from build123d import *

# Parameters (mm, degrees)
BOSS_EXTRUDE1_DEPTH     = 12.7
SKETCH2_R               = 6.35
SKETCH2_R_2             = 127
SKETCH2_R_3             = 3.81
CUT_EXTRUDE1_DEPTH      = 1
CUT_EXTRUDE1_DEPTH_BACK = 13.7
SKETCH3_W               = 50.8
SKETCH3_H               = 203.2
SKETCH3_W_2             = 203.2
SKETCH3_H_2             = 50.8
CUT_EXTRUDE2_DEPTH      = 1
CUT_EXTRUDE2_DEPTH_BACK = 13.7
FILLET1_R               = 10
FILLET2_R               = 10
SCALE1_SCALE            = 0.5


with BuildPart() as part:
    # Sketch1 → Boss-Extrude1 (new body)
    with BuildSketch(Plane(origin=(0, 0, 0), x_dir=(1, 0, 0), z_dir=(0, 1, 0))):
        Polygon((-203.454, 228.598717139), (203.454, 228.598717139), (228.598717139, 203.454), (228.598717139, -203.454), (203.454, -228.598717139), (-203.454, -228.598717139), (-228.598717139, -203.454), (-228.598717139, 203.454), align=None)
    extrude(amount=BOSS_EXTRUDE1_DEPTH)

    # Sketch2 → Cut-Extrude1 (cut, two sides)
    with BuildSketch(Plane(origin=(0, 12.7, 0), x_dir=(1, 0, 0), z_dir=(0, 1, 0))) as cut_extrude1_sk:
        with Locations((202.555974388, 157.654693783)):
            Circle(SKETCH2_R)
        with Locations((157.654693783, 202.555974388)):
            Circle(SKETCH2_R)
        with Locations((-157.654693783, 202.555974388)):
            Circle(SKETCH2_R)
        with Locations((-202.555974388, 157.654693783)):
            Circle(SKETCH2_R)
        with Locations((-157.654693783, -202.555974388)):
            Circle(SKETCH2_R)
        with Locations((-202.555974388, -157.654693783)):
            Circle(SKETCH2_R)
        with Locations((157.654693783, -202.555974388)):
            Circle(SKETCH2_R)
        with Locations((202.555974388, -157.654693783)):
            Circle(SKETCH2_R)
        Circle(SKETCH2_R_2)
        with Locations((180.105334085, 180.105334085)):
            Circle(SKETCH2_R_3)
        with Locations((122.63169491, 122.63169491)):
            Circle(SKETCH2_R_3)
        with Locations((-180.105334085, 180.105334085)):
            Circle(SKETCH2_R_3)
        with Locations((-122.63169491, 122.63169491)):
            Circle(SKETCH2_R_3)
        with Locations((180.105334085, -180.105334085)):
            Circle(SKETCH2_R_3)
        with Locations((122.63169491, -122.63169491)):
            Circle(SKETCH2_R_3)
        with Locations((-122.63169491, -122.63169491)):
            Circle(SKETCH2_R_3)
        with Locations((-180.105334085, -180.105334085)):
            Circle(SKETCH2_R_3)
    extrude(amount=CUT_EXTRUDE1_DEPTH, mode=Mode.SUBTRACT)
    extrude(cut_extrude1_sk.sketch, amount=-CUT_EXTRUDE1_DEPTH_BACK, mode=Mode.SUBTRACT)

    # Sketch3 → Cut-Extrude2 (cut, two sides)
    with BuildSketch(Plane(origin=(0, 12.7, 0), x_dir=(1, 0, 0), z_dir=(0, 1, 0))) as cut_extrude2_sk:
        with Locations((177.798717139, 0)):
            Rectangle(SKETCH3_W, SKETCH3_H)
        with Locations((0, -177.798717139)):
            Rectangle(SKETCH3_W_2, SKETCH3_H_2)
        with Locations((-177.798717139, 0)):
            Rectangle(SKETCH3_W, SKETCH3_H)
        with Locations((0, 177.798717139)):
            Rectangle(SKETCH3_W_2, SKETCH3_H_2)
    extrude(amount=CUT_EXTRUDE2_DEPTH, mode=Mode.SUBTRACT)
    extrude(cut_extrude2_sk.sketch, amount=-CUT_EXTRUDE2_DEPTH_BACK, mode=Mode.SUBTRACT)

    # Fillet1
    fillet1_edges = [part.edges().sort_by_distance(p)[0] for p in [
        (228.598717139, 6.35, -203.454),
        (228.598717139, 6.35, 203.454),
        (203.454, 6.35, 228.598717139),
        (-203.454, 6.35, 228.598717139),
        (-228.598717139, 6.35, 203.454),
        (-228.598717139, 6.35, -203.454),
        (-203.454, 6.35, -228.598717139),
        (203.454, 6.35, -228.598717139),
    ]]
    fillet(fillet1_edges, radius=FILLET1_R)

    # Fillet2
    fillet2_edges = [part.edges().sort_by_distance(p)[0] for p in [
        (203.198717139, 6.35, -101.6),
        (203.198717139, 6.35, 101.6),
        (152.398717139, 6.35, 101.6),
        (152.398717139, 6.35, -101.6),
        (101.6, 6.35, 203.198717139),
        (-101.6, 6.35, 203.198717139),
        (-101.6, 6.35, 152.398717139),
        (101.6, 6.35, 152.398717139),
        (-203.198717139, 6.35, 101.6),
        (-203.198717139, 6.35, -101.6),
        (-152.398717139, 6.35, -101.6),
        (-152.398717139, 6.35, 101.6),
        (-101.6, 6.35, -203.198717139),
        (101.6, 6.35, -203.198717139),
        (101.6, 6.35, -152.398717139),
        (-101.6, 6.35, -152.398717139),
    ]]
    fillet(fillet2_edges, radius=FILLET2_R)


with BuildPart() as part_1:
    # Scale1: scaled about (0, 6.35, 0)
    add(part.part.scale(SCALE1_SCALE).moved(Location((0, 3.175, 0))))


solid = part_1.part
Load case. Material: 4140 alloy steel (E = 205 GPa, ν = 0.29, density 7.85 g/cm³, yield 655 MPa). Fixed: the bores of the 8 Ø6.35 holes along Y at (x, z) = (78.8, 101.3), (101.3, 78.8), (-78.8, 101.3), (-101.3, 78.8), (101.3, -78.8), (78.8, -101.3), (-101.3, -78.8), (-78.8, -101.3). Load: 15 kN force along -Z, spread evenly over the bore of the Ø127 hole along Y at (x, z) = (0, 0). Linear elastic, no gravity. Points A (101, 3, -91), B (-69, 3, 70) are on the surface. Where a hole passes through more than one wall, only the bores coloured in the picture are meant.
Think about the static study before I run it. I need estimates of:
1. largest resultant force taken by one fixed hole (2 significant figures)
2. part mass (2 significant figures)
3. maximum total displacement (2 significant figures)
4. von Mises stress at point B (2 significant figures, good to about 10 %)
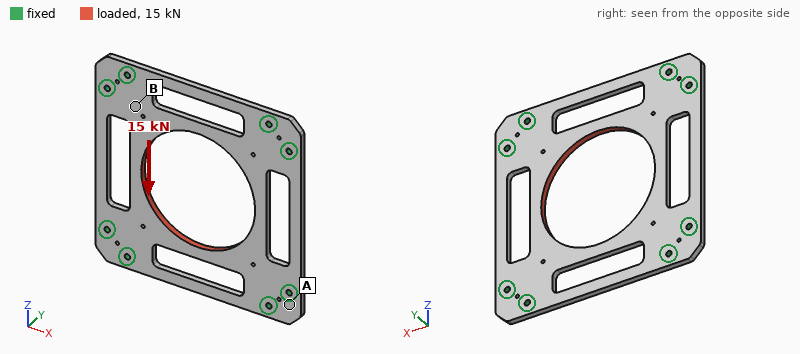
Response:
4.6 kN
1.4 kg
36 µm
14 MPa
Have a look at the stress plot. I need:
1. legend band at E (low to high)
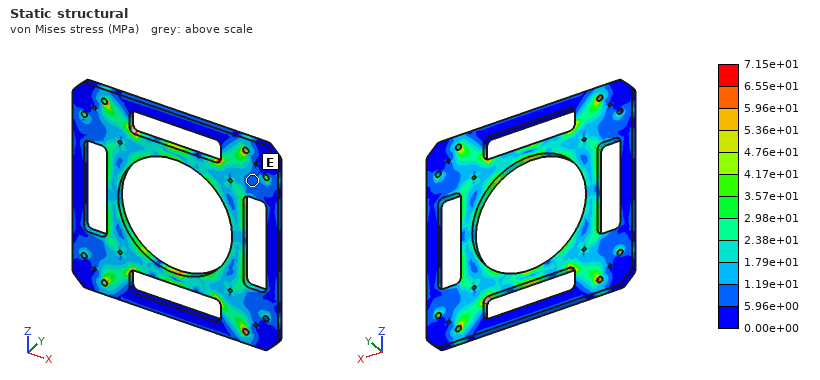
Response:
5.96e+00 to 1.19e+01 MPa
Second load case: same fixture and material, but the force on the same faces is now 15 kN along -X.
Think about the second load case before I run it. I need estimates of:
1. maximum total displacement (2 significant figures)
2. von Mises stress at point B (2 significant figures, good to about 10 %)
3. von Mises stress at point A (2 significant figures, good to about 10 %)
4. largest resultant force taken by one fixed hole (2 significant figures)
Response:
36 µm
14 MPa
7.6 MPa
4.7 kN
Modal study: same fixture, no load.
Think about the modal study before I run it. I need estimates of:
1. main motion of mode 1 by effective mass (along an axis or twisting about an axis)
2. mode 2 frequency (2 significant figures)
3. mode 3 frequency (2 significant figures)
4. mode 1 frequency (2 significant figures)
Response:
along Y
1400 Hz
1400 Hz
1100 Hz
